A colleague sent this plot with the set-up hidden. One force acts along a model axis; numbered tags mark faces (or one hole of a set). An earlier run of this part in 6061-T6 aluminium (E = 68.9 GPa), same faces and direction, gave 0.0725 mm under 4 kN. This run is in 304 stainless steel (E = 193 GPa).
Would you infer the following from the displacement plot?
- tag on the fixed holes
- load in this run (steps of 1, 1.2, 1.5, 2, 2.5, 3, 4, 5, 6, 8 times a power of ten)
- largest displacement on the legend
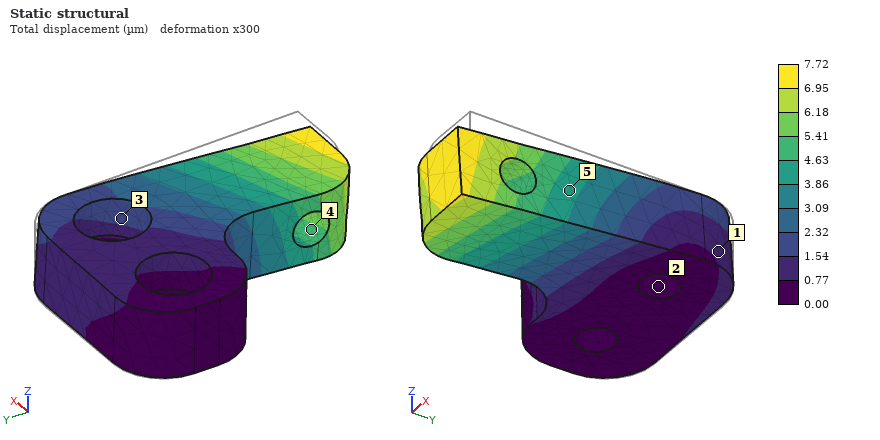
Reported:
2
1.2 kN
7.72 µm
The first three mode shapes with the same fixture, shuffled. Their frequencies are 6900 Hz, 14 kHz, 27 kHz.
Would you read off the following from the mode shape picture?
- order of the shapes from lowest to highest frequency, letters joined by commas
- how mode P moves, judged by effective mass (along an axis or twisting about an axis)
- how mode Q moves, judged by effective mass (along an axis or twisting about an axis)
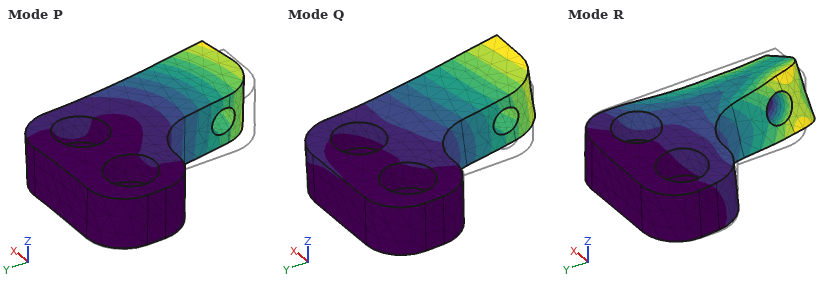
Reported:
Q, P, R
along X
along Z
